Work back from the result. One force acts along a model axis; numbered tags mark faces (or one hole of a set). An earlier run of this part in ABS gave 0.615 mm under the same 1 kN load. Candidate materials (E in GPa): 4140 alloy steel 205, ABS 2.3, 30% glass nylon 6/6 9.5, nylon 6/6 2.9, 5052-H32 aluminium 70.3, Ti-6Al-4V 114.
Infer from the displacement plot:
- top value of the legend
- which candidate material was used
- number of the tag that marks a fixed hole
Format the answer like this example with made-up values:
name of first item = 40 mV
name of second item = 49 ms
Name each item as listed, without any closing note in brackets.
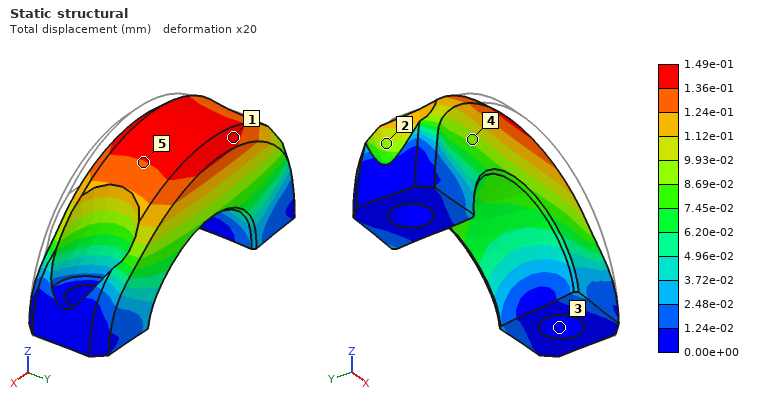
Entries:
top value of the legend = 1.49e-01 mm
which candidate material was used = 30% glass nylon 6/6
number of the tag that marks a fixed hole = 3
